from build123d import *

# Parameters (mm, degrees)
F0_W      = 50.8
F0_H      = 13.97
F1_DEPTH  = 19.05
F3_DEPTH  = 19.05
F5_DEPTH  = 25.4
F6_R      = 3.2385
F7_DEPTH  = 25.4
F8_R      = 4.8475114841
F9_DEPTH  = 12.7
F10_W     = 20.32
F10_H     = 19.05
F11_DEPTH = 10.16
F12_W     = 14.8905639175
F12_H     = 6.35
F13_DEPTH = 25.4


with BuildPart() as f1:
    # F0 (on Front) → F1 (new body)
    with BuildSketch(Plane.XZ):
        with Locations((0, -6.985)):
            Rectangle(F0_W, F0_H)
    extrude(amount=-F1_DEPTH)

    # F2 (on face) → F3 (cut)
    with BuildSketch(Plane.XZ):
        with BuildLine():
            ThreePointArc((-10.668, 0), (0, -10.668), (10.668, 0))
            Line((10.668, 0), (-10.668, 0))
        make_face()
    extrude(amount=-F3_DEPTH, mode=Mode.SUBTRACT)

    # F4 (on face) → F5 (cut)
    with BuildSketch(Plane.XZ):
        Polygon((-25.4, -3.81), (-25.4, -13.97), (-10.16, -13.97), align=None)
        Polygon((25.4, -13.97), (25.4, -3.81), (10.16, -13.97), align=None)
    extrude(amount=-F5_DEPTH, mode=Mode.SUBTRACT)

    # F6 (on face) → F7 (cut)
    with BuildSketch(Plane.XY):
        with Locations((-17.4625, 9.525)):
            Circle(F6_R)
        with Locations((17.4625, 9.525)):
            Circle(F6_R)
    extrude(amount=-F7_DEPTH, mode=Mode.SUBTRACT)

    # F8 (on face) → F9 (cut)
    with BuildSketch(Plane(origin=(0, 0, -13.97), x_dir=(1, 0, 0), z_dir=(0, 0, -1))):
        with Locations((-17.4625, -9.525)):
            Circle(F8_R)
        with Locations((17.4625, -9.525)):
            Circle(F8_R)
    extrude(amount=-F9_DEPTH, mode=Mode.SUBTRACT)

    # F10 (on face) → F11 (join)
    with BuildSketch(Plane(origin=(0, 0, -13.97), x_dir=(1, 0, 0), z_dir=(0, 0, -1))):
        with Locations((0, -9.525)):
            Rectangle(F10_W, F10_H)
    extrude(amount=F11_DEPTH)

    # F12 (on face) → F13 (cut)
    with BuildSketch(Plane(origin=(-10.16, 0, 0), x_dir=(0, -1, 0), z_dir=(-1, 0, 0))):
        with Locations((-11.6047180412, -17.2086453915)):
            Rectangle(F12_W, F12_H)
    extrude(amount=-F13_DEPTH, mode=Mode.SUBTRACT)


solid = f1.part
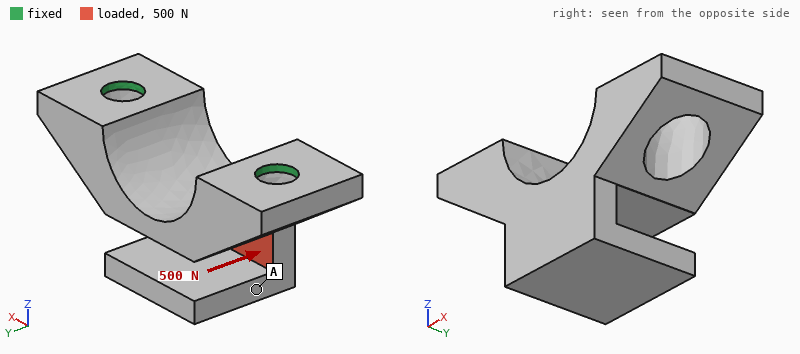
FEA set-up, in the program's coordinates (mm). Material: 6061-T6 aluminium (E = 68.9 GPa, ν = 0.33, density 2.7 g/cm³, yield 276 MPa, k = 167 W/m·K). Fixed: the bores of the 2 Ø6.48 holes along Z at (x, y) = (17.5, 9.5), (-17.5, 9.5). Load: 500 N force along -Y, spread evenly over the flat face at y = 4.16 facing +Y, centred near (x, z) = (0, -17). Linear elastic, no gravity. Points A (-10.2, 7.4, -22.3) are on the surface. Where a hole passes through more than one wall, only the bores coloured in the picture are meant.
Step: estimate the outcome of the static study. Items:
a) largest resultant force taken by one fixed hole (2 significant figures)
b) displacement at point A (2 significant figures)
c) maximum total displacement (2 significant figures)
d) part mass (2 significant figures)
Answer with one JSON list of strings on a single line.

["250 N", "77 µm", "96 µm", "21 g"]
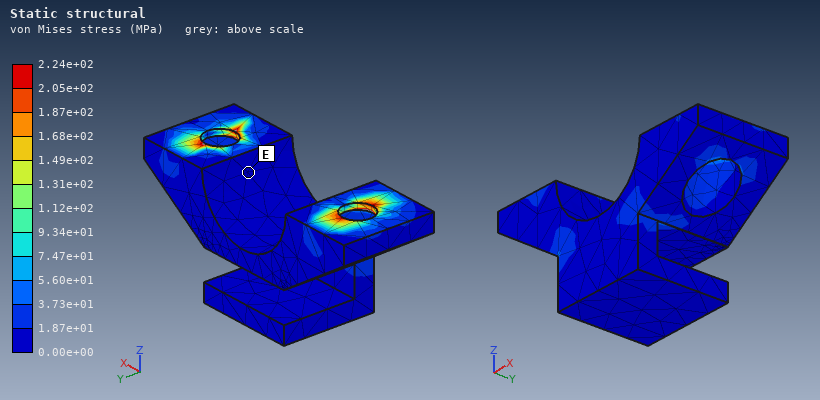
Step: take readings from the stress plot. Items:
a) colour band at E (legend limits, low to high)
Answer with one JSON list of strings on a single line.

["0.00e+00 to 1.87e+01 MPa"]
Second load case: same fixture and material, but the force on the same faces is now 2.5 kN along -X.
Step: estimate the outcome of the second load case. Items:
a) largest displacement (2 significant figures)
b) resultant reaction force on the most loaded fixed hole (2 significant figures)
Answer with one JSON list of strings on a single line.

["53 µm", "1.8 kN"]
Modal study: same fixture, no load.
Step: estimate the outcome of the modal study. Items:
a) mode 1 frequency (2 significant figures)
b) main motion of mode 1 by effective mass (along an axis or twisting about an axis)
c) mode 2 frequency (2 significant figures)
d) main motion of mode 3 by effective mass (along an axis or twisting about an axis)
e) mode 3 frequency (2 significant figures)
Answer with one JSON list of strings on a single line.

["3900 Hz", "along Y", "7000 Hz", "along X", "8400 Hz"]
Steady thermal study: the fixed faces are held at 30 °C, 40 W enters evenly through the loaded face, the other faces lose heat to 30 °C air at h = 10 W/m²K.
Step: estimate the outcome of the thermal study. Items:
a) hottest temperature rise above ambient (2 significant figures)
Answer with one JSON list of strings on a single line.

["43 K"]
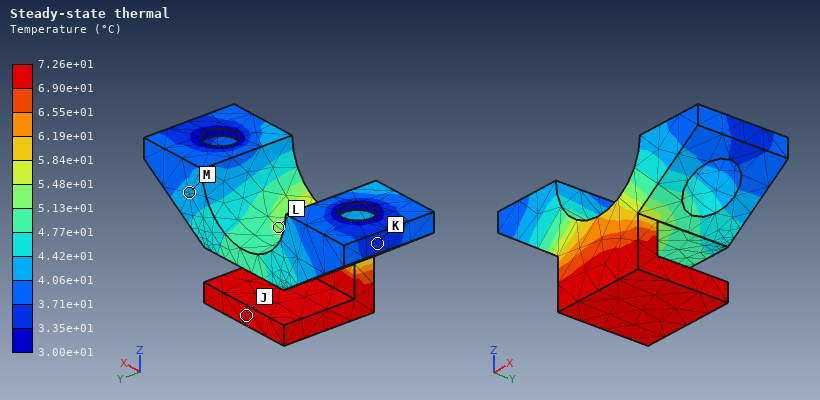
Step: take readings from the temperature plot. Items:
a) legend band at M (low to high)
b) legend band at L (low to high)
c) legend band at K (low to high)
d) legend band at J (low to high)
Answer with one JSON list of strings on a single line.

["4.06e+01 to 4.42e+01 °C", "5.13e+01 to 5.48e+01 °C", "3.35e+01 to 3.71e+01 °C", "6.90e+01 to 7.26e+01 °C"]
